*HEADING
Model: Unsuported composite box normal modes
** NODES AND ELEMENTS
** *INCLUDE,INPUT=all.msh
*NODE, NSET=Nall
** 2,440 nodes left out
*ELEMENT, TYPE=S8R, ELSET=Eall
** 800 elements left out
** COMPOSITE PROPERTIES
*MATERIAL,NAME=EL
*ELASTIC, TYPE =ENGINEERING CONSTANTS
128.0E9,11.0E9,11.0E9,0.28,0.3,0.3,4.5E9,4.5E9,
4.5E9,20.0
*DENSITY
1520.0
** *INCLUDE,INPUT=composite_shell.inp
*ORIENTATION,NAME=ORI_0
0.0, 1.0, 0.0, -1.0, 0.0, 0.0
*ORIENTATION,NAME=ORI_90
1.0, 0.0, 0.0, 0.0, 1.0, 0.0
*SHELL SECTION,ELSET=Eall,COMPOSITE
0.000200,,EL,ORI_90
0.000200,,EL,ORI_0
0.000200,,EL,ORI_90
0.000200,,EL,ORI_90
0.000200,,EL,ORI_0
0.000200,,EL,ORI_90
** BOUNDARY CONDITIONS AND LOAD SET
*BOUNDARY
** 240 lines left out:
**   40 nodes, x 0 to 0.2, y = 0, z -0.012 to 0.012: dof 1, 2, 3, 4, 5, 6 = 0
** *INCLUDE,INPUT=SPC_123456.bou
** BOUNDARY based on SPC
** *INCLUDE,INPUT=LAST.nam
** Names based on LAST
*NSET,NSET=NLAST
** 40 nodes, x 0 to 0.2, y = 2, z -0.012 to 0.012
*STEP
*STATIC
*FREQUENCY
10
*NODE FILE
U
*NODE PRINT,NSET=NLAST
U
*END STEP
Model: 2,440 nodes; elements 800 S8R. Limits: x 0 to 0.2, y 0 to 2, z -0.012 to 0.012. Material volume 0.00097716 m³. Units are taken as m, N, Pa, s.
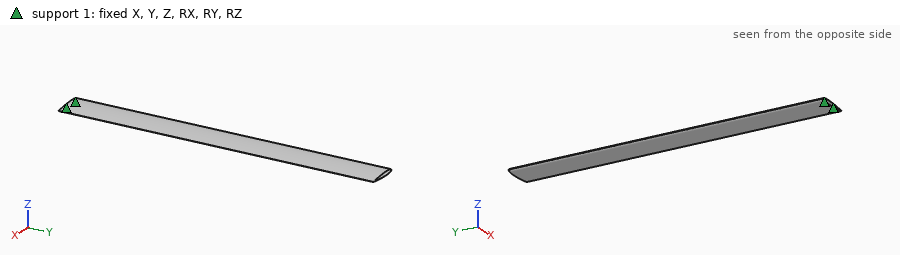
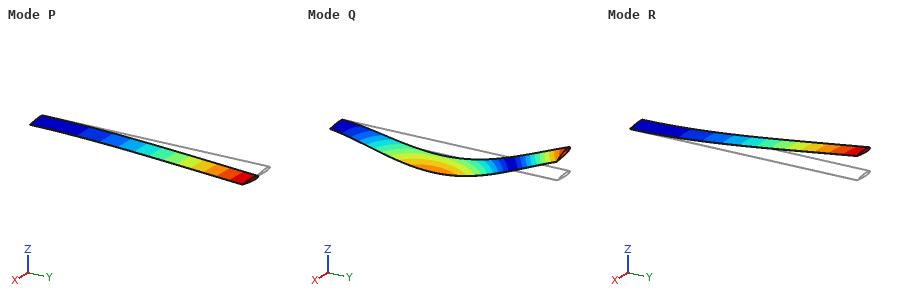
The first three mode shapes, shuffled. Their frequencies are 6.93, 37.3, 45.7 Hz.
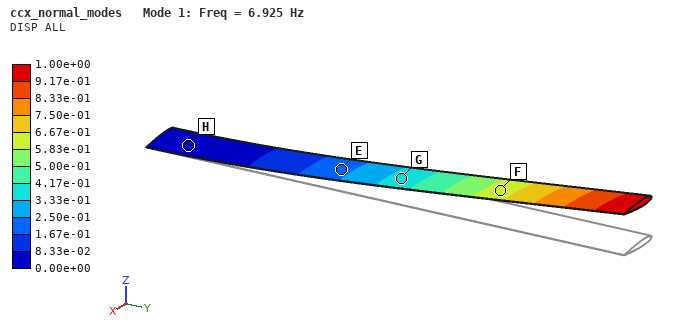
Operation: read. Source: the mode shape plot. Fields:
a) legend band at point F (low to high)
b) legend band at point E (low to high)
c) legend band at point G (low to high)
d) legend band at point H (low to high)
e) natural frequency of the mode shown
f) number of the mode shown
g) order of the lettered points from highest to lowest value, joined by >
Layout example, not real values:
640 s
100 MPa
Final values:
5.83e-01 to 6.67e-01
1.67e-01 to 2.50e-01
3.33e-01 to 4.17e-01
0.00e+00 to 8.33e-02
6.925 Hz
1
F > G > E > H
